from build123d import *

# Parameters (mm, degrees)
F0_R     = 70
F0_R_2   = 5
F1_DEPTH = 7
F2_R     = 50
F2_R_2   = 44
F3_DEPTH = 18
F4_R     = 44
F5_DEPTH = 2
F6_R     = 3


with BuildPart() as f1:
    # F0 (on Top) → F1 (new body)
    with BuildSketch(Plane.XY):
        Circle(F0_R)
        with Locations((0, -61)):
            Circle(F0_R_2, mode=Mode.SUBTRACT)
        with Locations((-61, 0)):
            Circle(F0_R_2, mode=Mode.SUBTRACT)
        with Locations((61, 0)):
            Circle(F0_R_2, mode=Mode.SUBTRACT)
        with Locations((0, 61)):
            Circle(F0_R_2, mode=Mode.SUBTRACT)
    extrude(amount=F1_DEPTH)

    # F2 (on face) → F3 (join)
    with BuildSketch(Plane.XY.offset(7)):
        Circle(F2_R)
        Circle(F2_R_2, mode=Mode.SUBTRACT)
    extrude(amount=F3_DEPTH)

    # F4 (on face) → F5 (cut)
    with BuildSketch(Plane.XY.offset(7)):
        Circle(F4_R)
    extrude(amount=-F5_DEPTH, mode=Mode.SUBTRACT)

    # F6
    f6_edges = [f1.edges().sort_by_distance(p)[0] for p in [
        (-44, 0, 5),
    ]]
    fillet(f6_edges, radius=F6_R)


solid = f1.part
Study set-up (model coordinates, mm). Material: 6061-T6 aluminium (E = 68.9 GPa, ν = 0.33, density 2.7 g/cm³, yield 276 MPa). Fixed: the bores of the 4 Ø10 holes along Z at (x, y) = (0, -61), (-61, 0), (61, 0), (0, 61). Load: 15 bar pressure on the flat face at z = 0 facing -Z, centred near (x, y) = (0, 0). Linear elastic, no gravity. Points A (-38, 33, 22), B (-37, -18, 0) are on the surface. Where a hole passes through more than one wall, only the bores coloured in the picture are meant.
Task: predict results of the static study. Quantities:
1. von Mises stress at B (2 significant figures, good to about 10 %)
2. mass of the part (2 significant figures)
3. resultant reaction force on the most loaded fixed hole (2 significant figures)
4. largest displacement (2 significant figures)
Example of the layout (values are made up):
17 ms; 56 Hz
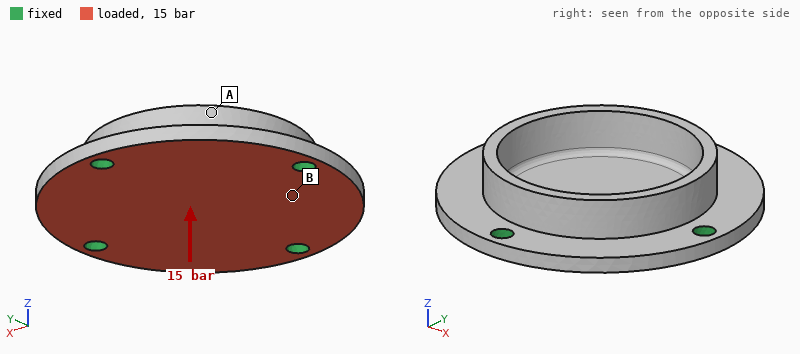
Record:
61 MPa; 340 g; 5.7 kN; 0.20 mm
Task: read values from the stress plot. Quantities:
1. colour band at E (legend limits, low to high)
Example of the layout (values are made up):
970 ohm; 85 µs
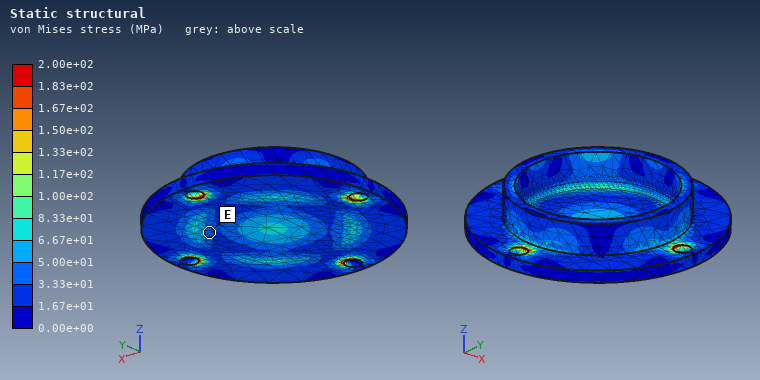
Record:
3.33e+01 to 5.00e+01 MPa
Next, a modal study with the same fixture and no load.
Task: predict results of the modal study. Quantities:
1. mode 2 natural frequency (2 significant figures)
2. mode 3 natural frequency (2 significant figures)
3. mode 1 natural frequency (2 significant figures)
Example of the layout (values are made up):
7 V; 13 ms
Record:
4600 Hz; 5400 Hz; 4500 Hz
